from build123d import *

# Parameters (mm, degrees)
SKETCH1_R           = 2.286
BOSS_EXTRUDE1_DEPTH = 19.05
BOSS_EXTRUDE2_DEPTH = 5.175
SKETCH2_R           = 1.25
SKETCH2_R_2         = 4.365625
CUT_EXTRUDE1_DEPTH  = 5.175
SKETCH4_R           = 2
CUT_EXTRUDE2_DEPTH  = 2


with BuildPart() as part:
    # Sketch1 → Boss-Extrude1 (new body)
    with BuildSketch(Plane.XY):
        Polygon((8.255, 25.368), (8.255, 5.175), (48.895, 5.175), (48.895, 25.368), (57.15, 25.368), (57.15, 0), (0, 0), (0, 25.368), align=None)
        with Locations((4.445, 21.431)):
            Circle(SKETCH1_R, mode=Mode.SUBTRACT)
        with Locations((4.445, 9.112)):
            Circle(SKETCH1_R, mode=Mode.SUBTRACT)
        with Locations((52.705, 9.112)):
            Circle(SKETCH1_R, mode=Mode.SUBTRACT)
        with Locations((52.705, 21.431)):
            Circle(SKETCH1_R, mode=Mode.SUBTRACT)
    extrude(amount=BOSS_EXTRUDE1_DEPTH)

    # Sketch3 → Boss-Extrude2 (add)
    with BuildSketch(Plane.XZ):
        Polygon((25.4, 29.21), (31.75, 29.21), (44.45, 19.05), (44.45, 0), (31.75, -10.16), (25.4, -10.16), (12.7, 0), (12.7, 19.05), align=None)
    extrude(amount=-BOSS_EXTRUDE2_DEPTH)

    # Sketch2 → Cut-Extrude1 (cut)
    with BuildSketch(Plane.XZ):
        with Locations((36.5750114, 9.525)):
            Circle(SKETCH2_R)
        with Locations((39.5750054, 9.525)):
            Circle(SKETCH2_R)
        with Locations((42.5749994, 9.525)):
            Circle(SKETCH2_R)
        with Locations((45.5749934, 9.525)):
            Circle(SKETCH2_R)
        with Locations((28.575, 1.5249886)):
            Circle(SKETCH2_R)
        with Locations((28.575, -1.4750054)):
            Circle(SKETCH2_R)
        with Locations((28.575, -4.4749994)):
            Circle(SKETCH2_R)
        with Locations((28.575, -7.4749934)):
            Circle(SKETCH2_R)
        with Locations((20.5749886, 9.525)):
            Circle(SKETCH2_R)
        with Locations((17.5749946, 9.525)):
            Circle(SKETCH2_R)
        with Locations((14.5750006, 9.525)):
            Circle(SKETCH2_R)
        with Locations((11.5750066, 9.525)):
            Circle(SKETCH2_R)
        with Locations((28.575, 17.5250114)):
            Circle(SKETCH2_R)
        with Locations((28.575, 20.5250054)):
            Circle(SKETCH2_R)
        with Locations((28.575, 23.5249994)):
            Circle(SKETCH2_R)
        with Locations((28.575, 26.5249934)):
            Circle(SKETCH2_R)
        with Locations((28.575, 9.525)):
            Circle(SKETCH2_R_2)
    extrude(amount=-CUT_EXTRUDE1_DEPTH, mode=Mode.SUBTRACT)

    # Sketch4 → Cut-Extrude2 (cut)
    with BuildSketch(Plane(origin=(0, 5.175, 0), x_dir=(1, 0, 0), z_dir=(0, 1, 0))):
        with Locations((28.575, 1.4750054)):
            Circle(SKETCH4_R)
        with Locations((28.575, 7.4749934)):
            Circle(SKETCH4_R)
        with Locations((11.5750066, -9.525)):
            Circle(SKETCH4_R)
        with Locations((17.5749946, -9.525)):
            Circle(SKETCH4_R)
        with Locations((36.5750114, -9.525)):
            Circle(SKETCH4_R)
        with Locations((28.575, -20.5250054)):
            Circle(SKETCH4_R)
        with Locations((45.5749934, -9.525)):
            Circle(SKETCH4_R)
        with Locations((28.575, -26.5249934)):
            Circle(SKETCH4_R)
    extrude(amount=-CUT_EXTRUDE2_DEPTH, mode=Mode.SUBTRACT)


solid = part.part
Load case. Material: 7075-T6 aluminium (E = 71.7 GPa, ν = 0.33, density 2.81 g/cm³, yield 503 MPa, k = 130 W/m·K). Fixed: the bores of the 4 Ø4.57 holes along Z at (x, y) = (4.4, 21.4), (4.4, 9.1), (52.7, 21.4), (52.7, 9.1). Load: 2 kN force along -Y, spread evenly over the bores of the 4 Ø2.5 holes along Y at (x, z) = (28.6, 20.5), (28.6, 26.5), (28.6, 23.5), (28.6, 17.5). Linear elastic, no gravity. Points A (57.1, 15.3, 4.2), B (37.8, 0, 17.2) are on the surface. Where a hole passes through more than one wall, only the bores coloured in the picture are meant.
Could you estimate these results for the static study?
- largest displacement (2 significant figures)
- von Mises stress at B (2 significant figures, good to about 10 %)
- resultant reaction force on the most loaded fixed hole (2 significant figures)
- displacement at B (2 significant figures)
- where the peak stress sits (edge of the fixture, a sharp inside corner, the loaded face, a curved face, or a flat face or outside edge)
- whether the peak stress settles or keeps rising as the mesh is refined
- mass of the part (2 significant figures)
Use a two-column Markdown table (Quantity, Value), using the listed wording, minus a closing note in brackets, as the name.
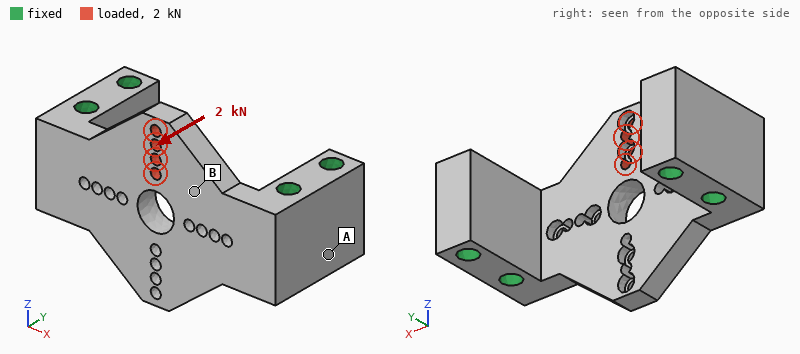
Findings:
| Quantity | Value |
|---|---|
| largest displacement | 0.30 mm |
| von Mises stress at B | 130 MPa |
| resultant reaction force on the most loaded fixed hole | 1.5 kN |
| displacement at B | 0.11 mm |
| where the peak stress sits | a sharp inside corner |
| whether the peak stress settles or keeps rising as the mesh is refined | keeps rising |
| mass of the part | 33 g |
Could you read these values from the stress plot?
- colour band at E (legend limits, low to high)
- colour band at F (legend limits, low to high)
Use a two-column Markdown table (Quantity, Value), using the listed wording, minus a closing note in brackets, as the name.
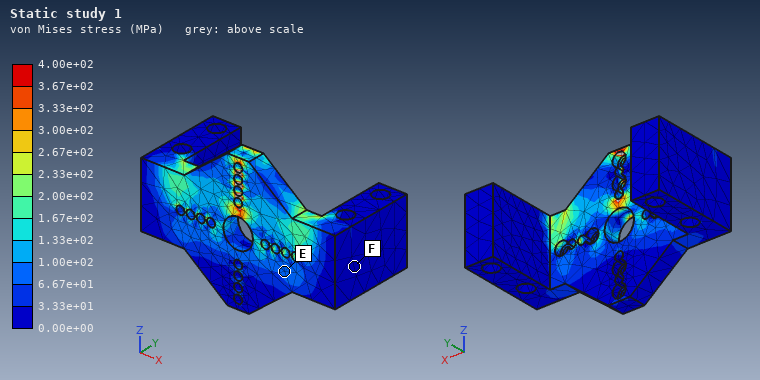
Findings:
| Quantity | Value |
|---|---|
| colour band at E | 6.67e+01 to 1.00e+02 MPa |
| colour band at F | 0.00e+00 to 3.33e+01 MPa |
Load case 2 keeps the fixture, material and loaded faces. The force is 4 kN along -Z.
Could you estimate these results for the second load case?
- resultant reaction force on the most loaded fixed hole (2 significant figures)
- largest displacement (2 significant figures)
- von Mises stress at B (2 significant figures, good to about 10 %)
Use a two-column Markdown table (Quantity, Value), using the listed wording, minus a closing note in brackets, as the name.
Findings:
| Quantity | Value |
|---|---|
| resultant reaction force on the most loaded fixed hole | 2.1 kN |
| largest displacement | 50 µm |
| von Mises stress at B | 49 MPa |
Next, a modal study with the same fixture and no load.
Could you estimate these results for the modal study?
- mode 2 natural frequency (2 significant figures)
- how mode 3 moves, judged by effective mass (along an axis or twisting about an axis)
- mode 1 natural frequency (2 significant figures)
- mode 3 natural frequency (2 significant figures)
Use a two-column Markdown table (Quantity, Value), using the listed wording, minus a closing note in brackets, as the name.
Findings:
| Quantity | Value |
|---|---|
| mode 2 natural frequency | 8900 Hz |
| how mode 3 moves, judged by effective mass | along Z |
| mode 1 natural frequency | 8600 Hz |
| mode 3 natural frequency | 19 kHz |
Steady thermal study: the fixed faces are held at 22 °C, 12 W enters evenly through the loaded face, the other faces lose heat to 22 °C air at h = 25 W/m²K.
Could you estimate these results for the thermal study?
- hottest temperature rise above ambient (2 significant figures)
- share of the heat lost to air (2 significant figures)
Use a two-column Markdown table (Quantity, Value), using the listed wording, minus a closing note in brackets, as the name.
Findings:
| Quantity | Value |
|---|---|
| hottest temperature rise above ambient | 19 K |
| share of the heat lost to air | 4.9 % |
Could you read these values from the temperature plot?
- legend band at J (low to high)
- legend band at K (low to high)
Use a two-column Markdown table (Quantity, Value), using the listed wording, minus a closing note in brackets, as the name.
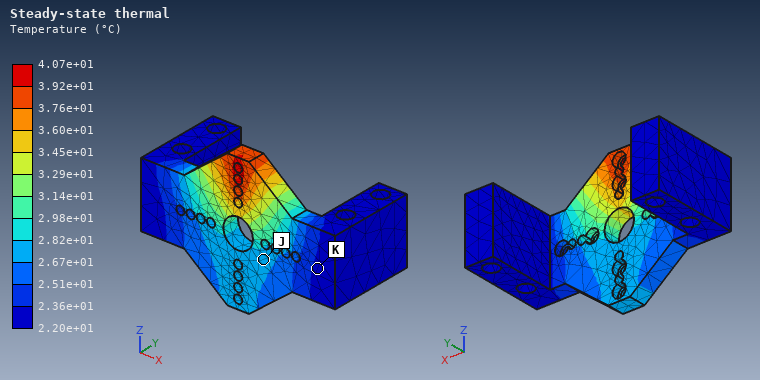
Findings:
| Quantity | Value |
|---|---|
| legend band at J | 2.67e+01 to 2.82e+01 °C |
| legend band at K | 2.20e+01 to 2.36e+01 °C |
